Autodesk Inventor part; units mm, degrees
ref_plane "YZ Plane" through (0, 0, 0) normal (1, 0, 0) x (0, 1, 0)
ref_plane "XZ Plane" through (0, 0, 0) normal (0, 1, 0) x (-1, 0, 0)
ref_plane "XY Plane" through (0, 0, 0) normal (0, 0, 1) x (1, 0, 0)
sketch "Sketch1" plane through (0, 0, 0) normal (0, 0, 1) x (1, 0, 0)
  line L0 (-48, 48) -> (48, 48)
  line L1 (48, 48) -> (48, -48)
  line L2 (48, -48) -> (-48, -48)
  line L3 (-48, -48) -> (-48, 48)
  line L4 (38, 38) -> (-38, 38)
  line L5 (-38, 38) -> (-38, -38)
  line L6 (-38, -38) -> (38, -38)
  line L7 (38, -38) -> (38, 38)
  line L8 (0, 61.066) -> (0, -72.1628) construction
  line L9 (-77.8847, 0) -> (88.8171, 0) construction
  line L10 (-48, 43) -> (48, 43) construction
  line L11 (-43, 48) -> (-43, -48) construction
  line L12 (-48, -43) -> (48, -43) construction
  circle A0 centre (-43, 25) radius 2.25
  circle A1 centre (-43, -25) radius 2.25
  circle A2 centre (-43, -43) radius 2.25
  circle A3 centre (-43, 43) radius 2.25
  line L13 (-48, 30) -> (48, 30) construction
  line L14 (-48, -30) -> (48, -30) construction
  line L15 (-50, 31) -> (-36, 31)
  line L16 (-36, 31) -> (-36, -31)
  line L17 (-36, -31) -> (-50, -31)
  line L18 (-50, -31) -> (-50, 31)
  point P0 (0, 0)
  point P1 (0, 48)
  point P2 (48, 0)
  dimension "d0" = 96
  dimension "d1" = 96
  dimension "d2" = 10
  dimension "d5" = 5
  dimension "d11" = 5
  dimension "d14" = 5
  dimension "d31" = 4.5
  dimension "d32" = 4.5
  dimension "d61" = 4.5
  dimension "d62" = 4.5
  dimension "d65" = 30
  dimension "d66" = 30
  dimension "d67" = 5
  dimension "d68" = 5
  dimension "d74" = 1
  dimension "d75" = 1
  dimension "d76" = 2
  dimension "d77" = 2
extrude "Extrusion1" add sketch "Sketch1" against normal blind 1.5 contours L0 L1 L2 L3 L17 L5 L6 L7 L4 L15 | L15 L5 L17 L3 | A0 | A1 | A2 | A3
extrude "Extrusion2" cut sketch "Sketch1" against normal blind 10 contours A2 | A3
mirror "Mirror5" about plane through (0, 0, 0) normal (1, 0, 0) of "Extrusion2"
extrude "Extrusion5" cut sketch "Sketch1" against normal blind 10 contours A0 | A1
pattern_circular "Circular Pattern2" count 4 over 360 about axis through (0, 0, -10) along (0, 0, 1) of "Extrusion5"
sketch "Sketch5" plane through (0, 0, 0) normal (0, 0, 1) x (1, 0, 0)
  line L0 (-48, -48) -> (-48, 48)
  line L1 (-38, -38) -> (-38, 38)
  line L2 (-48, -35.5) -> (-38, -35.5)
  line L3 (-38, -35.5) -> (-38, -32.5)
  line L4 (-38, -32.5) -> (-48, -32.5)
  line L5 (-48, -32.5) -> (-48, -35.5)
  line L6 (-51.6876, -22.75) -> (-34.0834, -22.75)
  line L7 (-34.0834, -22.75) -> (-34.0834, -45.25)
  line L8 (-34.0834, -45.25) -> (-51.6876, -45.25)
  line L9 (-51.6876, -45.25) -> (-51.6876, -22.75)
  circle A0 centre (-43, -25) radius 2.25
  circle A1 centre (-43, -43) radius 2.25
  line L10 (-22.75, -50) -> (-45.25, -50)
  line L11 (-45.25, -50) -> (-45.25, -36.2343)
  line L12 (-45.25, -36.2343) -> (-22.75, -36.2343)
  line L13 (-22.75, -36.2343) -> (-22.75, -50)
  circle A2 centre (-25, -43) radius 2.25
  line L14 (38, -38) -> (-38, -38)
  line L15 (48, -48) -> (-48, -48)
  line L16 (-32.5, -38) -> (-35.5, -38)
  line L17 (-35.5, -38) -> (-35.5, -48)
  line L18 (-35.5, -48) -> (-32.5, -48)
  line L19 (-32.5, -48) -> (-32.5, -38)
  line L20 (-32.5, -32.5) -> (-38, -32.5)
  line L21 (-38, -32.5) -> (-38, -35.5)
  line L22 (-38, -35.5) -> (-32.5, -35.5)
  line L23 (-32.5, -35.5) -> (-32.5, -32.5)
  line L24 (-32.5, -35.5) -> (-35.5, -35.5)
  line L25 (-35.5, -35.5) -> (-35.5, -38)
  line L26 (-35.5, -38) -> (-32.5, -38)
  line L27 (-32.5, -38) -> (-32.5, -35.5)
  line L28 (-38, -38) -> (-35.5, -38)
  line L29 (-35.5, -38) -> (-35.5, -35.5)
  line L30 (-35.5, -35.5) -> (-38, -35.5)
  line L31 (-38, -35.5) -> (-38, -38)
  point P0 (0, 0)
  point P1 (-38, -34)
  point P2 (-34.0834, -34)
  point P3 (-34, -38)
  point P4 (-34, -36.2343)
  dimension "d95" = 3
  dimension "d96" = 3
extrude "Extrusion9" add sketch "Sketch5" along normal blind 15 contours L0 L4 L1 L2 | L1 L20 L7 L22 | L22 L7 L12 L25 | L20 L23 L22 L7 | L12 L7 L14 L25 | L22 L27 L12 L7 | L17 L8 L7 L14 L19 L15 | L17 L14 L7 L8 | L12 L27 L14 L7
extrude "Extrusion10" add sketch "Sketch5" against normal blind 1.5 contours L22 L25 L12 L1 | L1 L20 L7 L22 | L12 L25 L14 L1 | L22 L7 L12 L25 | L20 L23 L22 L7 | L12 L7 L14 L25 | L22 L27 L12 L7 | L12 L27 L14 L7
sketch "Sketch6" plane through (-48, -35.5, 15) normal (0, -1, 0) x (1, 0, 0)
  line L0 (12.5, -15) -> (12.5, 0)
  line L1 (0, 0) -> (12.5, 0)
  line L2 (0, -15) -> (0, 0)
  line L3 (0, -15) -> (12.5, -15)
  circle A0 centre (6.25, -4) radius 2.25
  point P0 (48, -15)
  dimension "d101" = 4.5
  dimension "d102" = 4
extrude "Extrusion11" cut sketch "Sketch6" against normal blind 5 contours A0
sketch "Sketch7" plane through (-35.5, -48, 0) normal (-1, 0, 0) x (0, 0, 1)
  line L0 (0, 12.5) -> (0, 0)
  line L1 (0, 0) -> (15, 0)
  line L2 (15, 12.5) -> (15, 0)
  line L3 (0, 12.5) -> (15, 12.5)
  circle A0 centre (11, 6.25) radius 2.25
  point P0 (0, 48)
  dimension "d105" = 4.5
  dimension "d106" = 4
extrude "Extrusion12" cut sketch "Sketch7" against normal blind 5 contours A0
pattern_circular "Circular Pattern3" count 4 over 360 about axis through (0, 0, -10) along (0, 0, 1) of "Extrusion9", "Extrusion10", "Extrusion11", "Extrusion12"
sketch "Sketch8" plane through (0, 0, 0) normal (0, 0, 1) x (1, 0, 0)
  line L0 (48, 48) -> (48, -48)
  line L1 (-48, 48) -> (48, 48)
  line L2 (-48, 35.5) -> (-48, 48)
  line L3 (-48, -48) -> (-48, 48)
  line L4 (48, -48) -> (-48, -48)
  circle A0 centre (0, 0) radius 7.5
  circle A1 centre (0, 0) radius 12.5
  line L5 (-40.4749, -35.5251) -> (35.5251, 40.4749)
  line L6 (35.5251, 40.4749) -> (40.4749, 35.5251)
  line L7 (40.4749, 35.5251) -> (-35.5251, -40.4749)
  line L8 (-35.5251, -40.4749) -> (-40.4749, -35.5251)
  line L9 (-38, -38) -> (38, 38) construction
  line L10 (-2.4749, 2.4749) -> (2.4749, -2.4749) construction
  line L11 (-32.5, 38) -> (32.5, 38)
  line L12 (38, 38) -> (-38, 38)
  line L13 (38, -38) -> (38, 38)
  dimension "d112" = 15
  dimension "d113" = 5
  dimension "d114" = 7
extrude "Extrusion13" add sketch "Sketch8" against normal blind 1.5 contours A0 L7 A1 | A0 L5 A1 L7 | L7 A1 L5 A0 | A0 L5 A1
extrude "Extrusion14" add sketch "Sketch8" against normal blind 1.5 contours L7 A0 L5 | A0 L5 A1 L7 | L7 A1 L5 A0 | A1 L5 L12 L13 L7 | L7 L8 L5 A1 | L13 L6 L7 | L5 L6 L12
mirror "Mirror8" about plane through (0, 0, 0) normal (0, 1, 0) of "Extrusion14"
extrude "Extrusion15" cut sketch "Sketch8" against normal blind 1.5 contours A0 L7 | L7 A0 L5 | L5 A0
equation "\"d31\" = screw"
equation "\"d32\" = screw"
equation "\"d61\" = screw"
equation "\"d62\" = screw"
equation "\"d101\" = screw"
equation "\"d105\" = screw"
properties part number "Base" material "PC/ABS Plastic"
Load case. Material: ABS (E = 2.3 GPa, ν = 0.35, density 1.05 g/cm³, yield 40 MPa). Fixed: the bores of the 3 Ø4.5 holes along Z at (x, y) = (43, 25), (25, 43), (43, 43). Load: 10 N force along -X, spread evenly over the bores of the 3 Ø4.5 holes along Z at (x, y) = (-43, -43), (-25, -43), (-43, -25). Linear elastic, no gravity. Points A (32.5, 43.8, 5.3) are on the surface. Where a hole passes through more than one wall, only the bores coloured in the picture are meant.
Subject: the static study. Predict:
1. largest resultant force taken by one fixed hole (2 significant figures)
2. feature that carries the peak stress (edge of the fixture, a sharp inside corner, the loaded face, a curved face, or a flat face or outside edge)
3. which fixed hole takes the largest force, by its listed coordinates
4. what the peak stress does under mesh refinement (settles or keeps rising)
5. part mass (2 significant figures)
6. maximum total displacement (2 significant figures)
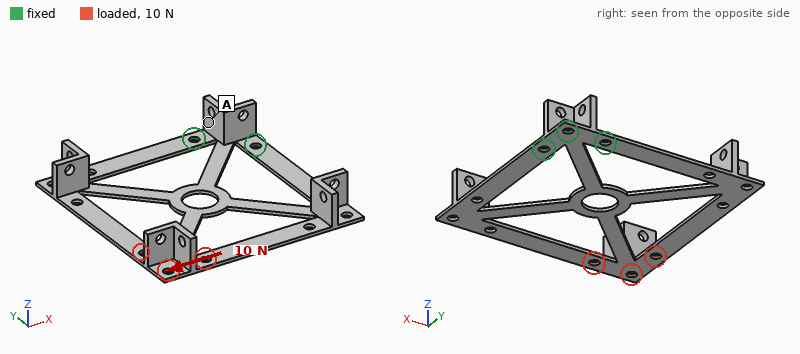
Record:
16 N
a sharp inside corner
(43, 25)
keeps rising
12 g
1.5 mm
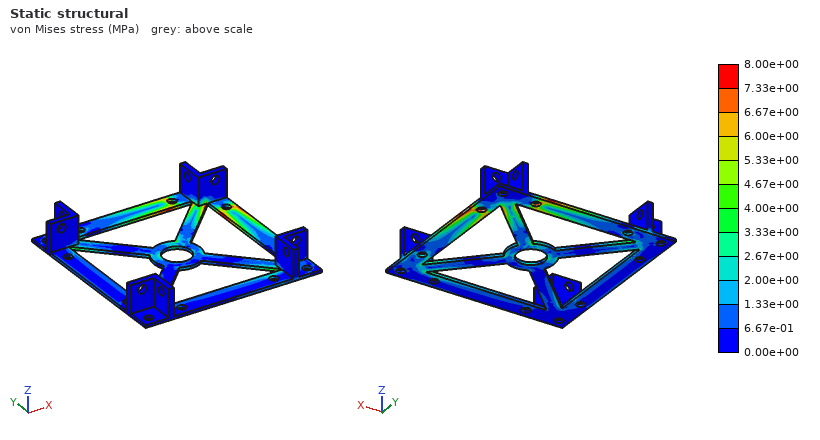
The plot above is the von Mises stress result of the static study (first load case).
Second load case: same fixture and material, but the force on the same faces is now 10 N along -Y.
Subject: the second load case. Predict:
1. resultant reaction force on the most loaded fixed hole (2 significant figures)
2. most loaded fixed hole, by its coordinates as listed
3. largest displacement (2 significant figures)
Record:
16 N
(25, 43)
1.5 mm
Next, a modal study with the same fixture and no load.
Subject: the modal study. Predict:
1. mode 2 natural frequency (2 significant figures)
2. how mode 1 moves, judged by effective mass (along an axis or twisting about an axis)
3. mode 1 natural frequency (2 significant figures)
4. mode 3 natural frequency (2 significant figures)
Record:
40 Hz
along Z
19 Hz
70 Hz
